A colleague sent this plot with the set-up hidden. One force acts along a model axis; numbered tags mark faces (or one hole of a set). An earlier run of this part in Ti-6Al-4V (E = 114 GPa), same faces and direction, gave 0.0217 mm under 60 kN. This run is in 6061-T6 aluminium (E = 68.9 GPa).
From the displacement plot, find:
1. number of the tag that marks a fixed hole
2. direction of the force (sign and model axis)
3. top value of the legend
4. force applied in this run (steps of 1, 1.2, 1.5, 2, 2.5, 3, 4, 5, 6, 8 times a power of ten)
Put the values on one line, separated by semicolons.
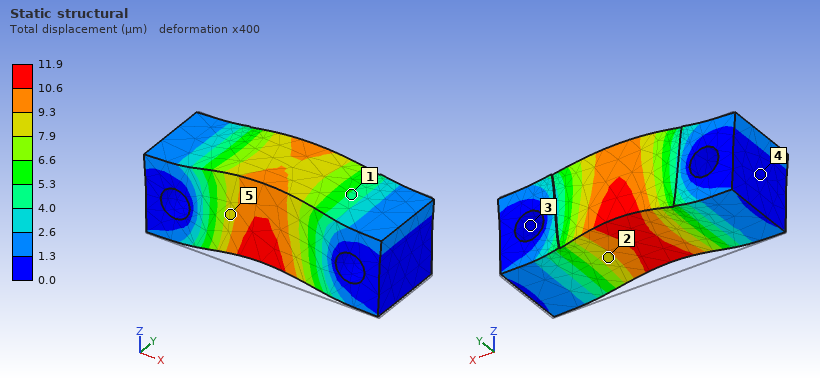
3; +Z; 11.9 µm; 20 kN
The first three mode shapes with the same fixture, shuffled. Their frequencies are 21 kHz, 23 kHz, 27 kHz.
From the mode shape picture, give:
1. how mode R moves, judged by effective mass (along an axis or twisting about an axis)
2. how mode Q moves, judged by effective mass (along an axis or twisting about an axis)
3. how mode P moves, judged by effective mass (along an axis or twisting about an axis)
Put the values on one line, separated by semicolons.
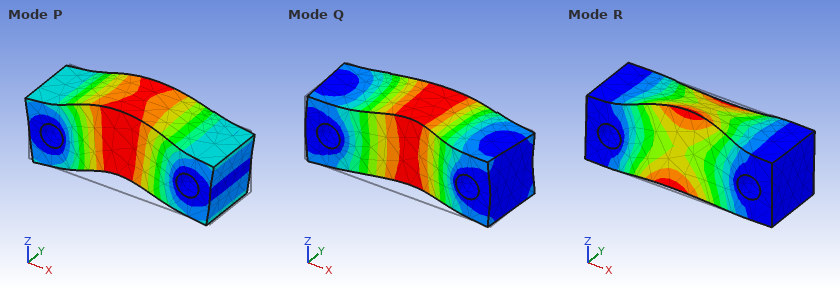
twisting about X; along Y; along Z
